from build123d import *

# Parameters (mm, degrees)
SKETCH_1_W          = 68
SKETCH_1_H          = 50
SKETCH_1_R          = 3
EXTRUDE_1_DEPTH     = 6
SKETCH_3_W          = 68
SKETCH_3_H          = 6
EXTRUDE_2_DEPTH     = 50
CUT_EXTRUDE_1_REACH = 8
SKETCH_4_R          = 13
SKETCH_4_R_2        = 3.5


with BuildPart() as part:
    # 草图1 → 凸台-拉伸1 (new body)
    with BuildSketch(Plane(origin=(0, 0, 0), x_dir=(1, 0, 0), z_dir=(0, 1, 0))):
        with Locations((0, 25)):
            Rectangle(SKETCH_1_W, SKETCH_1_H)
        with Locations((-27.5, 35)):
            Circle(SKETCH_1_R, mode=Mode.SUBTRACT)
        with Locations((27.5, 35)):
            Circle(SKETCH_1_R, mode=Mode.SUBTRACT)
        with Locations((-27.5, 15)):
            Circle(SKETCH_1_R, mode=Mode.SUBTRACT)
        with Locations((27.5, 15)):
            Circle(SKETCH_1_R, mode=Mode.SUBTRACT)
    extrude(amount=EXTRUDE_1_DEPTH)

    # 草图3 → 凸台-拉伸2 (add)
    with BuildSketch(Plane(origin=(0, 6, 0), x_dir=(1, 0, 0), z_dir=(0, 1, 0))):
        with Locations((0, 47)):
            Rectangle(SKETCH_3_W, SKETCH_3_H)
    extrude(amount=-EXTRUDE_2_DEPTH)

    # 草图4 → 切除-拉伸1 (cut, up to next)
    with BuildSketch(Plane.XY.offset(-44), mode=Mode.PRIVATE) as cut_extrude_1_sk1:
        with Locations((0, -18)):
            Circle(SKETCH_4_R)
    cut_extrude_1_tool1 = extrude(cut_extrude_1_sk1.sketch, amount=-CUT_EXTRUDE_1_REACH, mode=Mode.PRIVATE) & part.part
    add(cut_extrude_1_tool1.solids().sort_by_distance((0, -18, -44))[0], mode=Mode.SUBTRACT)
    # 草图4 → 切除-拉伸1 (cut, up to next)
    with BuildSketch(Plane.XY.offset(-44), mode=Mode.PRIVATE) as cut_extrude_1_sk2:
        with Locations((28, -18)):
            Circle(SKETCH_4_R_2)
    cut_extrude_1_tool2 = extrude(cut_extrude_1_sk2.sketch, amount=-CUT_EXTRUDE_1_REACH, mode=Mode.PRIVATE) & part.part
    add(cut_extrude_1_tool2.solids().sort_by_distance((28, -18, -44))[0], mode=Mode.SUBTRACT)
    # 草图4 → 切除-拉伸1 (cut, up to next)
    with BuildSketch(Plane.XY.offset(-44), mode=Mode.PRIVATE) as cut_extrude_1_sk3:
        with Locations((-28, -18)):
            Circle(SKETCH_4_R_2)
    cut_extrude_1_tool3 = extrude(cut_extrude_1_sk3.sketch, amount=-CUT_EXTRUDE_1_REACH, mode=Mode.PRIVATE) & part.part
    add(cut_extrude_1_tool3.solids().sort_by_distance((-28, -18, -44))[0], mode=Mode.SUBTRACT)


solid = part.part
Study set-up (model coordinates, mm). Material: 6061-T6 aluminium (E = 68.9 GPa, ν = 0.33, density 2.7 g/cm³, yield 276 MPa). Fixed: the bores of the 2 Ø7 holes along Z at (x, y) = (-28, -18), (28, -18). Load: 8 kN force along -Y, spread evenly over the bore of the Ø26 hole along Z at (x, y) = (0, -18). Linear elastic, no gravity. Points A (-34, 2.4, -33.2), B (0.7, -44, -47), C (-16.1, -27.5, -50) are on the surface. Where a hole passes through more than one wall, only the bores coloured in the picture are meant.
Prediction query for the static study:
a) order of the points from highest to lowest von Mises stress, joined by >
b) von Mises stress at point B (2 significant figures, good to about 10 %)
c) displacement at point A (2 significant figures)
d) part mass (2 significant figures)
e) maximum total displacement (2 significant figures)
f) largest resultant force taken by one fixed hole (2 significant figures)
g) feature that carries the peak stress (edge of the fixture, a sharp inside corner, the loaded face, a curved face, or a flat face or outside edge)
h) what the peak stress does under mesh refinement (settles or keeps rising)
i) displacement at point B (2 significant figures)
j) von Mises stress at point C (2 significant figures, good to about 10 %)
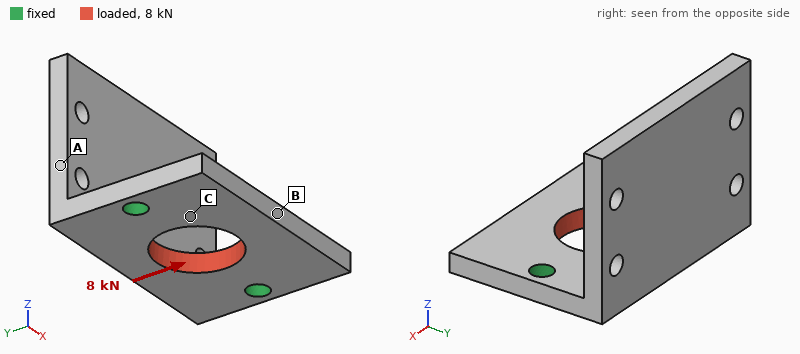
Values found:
B > C > A
43 MPa
3.3 µm
92 g
21 µm
4.0 kN
edge of the fixture
keeps rising
17 µm
27 MPa
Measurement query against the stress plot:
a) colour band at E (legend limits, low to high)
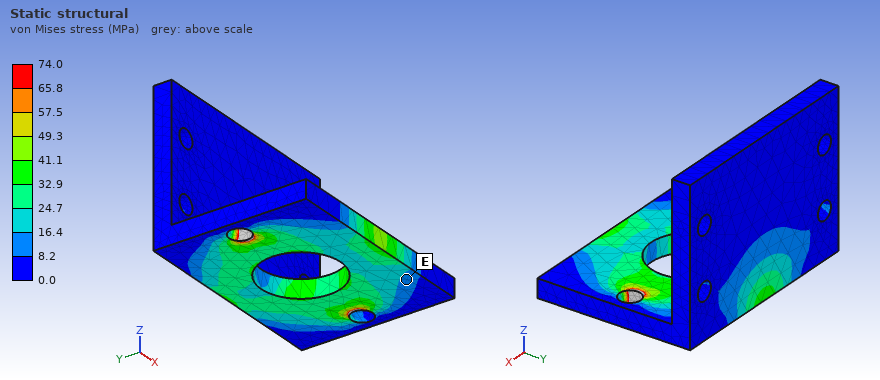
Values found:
8.2 to 16.4 MPa
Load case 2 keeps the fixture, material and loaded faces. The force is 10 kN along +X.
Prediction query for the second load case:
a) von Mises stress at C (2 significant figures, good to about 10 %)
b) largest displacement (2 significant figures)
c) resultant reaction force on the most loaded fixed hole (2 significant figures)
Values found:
35 MPa
17 µm
5.0 kN
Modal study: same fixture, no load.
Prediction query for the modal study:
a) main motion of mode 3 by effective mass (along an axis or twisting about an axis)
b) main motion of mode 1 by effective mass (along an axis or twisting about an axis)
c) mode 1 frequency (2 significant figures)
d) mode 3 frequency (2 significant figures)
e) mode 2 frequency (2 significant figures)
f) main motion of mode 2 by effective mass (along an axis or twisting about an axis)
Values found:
along Z
along Y
1200 Hz
4300 Hz
2900 Hz
along X
